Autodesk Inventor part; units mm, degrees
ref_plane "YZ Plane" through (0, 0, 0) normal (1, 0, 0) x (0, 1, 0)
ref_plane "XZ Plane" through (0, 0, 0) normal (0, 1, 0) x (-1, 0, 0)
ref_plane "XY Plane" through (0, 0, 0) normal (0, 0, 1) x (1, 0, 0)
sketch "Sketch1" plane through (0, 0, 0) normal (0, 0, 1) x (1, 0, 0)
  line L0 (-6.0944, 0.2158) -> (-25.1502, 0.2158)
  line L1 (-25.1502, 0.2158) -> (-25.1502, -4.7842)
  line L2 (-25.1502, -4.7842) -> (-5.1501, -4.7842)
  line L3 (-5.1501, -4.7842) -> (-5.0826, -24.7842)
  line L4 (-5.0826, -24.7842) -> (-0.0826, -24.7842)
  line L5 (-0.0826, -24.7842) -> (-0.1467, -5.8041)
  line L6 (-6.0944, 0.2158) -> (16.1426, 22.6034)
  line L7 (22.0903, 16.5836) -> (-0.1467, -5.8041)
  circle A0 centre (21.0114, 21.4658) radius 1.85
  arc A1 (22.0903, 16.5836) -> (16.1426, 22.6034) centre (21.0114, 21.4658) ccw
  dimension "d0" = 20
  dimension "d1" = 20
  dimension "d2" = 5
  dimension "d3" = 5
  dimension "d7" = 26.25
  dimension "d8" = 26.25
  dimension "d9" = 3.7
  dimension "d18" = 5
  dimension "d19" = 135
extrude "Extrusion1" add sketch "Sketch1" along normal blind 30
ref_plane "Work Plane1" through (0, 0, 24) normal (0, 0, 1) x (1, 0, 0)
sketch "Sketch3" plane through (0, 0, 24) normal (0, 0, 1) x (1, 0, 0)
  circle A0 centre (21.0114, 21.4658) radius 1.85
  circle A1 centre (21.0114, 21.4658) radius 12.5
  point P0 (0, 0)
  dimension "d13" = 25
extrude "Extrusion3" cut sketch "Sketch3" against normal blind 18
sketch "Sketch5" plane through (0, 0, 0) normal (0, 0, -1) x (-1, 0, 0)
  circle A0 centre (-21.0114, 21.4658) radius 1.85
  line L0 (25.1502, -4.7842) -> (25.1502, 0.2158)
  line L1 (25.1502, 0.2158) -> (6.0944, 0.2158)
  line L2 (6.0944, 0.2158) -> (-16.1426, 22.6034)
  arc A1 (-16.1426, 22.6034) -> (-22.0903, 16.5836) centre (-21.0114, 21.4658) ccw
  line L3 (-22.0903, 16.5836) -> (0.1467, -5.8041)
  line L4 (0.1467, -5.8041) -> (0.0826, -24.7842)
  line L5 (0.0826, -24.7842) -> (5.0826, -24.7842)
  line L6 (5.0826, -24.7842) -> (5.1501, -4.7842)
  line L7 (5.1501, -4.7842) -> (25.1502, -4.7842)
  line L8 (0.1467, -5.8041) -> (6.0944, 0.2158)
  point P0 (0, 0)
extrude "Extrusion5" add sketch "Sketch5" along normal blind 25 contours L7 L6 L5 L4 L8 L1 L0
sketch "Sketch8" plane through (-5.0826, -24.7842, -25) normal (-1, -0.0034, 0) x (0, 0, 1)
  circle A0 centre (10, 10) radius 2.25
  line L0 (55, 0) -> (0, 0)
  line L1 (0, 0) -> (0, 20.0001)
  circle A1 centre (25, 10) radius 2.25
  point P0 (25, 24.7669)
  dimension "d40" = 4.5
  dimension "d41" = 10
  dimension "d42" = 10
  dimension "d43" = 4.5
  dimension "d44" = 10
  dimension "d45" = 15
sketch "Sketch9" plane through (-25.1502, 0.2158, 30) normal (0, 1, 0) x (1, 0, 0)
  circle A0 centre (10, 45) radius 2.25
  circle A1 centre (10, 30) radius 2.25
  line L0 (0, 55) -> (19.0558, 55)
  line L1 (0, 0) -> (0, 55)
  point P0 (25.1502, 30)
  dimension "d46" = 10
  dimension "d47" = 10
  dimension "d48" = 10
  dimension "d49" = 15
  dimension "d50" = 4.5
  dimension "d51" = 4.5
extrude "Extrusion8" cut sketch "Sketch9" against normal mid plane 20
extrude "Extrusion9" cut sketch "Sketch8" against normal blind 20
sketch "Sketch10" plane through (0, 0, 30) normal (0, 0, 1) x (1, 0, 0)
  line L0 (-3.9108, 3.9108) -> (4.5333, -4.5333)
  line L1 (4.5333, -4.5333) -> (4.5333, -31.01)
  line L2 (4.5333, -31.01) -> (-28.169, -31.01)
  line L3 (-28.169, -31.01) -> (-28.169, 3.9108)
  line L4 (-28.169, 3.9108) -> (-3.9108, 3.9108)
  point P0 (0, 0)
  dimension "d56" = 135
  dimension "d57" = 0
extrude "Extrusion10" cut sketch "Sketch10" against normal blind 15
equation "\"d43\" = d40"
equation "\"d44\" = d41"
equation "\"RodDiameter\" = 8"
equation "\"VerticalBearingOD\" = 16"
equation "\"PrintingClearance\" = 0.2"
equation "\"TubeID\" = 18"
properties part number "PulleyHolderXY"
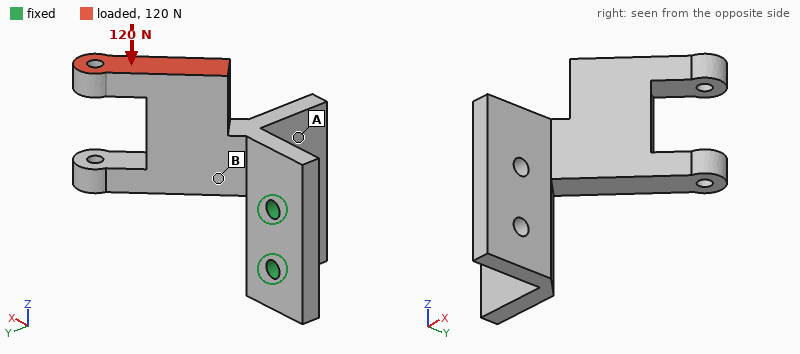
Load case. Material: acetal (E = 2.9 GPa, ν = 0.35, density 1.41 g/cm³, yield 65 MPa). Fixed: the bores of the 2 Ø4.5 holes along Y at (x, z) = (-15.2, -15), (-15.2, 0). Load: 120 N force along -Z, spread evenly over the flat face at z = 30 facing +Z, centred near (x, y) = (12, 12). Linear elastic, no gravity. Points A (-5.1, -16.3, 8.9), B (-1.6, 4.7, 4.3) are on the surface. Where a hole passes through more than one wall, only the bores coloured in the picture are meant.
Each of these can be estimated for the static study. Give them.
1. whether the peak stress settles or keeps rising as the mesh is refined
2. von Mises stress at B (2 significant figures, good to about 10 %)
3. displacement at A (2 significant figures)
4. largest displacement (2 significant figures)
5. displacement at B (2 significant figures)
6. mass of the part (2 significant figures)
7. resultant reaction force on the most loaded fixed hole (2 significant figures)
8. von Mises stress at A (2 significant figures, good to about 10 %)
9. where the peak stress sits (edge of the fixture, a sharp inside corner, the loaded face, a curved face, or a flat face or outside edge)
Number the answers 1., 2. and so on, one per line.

1. keeps rising
2. 4.4 MPa
3. 0.16 mm
4. 0.95 mm
5. 0.15 mm
6. 21 g
7. 180 N
8. 2.1 MPa
9. edge of the fixture
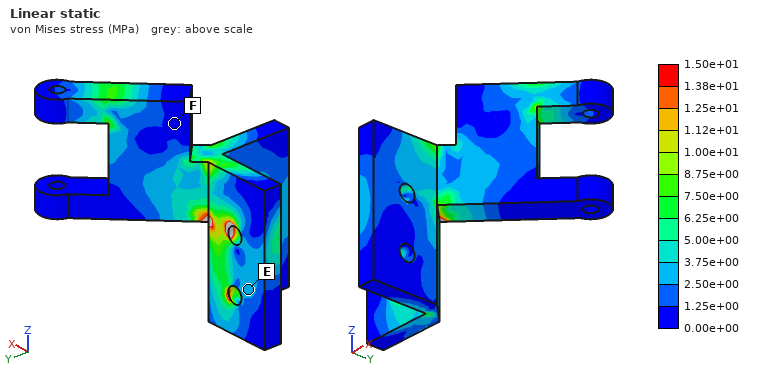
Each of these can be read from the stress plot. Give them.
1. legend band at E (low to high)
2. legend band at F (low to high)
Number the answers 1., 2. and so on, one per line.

1. 2.50e+00 to 3.75e+00 MPa
2. 0.00e+00 to 1.25e+00 MPa
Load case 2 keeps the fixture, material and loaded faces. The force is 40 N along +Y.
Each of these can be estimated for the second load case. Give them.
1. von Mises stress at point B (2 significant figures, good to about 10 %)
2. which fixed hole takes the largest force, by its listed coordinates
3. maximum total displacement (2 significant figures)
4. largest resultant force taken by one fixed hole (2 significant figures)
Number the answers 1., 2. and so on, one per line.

1. 4.4 MPa
2. (-15.2, 0)
3. 1.1 mm
4. 84 N
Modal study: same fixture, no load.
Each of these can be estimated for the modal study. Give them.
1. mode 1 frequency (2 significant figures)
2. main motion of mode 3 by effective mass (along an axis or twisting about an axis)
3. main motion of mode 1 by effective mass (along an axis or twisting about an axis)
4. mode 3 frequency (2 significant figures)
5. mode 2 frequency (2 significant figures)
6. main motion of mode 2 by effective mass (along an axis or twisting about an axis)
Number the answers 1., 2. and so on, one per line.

1. 470 Hz
2. along X
3. along Y
4. 1400 Hz
5. 910 Hz
6. along Z
